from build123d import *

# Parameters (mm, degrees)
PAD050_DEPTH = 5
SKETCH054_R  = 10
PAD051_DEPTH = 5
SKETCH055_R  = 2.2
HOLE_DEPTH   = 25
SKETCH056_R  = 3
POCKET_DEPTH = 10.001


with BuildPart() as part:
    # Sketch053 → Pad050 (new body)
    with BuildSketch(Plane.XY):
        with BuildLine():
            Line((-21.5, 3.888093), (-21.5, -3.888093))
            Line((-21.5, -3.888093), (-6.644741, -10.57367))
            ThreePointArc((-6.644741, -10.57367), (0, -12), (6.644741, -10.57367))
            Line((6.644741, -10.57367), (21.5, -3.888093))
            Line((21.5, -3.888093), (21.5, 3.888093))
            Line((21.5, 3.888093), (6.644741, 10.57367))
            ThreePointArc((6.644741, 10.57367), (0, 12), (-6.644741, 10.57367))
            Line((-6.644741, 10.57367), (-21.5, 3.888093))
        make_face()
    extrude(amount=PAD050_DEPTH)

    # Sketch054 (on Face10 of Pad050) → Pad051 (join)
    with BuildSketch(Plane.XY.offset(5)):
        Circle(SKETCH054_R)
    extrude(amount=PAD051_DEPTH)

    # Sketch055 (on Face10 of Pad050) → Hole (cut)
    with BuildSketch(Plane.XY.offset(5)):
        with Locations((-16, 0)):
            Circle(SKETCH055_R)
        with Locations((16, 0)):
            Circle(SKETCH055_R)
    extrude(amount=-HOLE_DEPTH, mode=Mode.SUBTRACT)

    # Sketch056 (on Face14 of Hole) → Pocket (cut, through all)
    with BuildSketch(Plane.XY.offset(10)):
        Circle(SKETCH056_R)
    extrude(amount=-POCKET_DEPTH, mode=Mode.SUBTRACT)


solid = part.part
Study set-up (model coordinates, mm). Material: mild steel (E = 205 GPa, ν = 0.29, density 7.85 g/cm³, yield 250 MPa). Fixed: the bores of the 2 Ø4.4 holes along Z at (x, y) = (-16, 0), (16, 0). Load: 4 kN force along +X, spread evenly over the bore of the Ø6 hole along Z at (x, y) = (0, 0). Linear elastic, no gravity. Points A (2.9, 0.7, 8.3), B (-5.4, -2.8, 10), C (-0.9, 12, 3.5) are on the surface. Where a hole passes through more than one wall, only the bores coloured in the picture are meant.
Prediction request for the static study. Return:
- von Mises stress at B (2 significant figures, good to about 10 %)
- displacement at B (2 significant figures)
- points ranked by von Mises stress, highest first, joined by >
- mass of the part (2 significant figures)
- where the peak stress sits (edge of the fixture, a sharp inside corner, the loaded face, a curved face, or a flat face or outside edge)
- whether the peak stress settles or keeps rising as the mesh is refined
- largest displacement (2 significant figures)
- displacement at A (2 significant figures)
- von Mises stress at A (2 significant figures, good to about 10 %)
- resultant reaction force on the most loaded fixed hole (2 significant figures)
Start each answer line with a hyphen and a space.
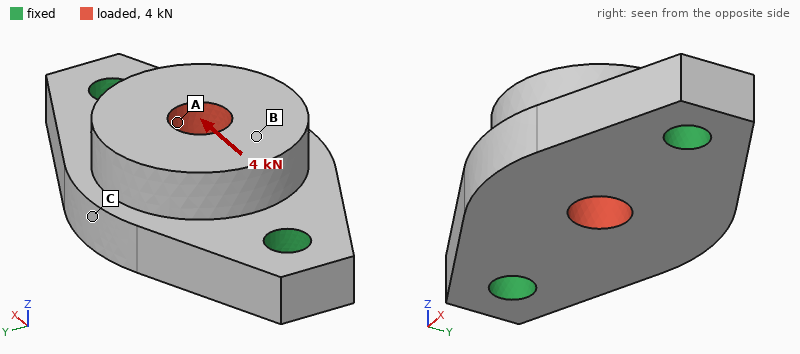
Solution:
- 15 MPa
- 2.4 µm
- A > B > C
- 38 g
- edge of the fixture
- keeps rising
- 2.7 µm
- 2.5 µm
- 23 MPa
- 2.0 kN
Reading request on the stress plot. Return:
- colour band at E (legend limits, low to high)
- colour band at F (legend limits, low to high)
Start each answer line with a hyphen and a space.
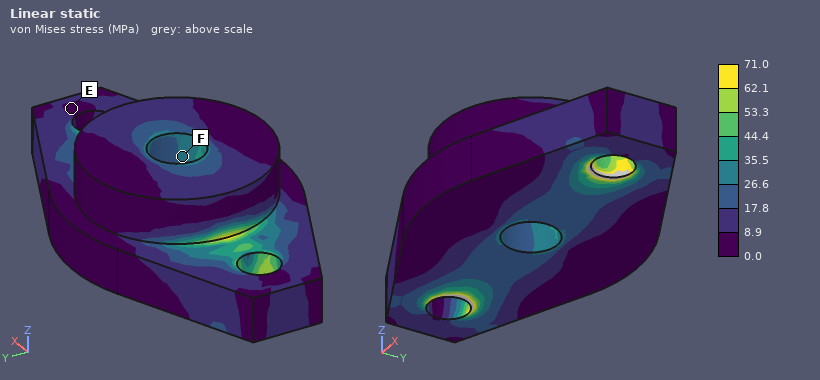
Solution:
- 0.0 to 8.9 MPa
- 26.6 to 35.5 MPa
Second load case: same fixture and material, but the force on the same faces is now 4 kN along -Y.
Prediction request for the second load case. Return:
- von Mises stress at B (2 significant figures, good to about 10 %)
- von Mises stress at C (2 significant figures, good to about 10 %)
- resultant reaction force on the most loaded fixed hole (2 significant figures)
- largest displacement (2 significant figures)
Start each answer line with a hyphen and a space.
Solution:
- 18 MPa
- 29 MPa
- 2.0 kN
- 13 µm
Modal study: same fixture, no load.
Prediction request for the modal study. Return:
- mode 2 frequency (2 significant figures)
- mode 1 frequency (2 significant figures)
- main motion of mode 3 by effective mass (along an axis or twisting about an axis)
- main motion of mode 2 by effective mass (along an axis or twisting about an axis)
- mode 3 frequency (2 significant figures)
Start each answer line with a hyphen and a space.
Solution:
- 21 kHz
- 15 kHz
- along Y
- along Z
- 32 kHz
